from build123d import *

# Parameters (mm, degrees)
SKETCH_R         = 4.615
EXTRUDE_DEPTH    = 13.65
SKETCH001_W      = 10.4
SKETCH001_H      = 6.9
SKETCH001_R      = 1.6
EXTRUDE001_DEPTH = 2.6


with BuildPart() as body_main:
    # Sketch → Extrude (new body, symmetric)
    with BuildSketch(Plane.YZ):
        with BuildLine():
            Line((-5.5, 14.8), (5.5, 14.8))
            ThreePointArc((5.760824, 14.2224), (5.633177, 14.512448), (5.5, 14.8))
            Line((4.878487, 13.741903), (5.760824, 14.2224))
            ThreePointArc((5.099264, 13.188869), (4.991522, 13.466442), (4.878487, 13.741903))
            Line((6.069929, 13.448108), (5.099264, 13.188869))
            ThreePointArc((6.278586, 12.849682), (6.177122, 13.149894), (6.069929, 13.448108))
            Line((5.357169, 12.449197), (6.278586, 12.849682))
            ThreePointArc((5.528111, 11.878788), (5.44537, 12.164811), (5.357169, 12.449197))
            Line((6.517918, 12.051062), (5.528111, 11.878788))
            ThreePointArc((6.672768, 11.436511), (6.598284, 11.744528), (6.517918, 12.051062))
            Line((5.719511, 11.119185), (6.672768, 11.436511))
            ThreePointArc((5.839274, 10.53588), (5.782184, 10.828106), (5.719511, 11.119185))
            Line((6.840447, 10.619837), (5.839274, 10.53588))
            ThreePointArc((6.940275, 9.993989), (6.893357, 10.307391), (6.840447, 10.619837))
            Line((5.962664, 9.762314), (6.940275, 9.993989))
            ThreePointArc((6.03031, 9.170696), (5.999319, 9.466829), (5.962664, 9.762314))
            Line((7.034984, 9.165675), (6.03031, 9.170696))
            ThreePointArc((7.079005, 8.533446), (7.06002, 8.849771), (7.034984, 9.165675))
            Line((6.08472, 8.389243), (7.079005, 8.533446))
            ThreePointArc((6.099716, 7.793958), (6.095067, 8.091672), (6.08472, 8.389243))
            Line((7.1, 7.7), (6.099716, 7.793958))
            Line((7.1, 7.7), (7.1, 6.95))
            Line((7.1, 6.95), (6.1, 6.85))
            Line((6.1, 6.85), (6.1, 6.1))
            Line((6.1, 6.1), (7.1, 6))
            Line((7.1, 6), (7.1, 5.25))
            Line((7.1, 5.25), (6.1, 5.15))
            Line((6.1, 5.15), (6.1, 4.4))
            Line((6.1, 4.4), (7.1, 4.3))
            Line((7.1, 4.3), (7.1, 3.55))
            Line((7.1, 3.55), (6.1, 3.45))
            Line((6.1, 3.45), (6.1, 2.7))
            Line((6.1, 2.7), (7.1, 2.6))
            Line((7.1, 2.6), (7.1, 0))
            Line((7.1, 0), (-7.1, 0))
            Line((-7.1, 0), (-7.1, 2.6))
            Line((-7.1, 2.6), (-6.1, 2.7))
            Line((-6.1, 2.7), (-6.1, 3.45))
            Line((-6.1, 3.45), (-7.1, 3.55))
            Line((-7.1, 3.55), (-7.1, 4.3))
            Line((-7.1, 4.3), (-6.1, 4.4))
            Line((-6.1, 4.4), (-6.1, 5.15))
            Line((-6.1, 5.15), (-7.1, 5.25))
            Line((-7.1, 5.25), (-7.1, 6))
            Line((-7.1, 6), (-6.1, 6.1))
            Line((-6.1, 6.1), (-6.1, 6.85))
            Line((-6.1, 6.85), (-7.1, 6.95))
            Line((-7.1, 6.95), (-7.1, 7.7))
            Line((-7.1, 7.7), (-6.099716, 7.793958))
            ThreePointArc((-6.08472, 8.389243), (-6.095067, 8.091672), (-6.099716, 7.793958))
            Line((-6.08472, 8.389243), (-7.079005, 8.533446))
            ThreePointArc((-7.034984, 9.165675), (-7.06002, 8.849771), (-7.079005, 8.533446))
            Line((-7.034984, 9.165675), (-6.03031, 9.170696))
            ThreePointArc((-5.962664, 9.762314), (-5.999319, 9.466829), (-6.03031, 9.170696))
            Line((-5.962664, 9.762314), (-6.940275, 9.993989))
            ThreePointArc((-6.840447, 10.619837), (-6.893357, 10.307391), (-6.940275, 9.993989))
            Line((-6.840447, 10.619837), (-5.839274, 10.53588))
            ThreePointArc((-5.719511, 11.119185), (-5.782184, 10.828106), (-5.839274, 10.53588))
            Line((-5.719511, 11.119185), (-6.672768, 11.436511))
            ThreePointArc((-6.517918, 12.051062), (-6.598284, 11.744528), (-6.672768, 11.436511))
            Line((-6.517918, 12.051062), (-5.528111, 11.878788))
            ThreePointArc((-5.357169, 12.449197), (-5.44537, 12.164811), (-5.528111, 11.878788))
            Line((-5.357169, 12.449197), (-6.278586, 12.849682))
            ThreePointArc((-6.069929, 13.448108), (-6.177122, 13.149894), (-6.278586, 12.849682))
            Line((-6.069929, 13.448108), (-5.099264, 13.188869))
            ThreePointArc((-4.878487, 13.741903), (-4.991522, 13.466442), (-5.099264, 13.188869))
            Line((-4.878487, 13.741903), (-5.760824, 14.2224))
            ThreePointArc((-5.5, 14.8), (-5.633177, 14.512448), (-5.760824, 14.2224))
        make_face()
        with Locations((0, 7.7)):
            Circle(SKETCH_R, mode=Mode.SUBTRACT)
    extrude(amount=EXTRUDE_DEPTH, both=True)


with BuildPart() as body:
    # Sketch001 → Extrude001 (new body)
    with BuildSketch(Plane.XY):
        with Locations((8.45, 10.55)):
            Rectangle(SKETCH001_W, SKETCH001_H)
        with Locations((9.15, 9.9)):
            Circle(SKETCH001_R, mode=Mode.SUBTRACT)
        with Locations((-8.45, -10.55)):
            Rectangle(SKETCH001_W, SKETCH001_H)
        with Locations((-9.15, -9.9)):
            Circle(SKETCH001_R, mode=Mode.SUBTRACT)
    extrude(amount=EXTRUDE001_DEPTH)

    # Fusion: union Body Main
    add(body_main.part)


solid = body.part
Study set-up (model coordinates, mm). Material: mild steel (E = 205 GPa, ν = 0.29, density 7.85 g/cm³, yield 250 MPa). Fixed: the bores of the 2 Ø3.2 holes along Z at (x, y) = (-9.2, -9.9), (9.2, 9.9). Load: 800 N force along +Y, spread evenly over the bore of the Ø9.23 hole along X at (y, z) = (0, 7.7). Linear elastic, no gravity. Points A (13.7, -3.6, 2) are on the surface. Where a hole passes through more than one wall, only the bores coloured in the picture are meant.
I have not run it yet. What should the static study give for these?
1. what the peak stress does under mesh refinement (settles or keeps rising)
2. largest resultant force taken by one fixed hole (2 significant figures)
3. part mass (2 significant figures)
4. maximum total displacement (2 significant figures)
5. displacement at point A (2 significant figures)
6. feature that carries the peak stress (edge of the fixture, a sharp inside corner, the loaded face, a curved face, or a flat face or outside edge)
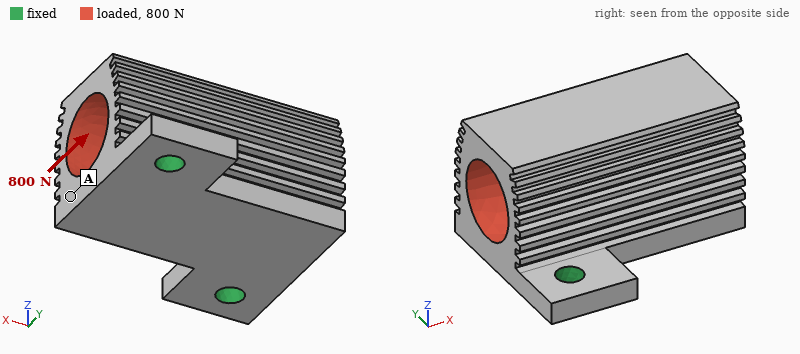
keeps rising
440 N
29 g
36 µm
20 µm
edge of the fixture
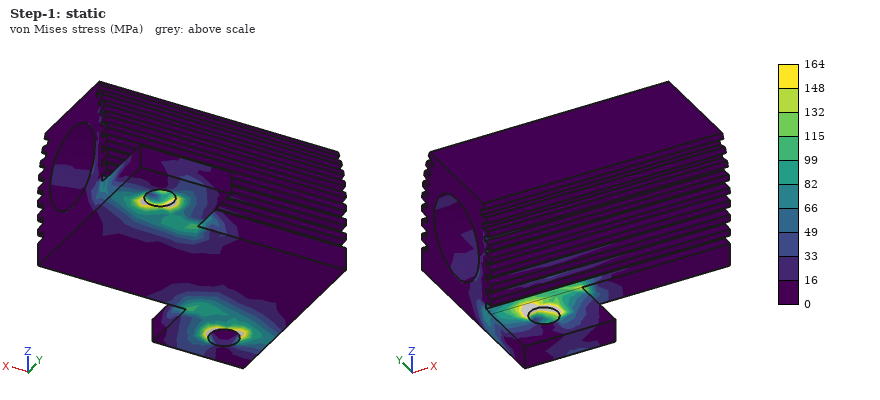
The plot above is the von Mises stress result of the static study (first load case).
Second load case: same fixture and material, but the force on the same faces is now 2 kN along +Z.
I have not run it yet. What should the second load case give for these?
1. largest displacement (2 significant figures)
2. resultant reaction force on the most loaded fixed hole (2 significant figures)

10 µm
1.0 kN
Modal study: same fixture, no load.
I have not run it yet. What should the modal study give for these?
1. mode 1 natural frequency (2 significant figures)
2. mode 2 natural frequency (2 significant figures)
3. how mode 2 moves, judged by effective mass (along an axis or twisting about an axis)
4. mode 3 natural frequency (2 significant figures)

4700 Hz
15 kHz
along Z
16 kHz
